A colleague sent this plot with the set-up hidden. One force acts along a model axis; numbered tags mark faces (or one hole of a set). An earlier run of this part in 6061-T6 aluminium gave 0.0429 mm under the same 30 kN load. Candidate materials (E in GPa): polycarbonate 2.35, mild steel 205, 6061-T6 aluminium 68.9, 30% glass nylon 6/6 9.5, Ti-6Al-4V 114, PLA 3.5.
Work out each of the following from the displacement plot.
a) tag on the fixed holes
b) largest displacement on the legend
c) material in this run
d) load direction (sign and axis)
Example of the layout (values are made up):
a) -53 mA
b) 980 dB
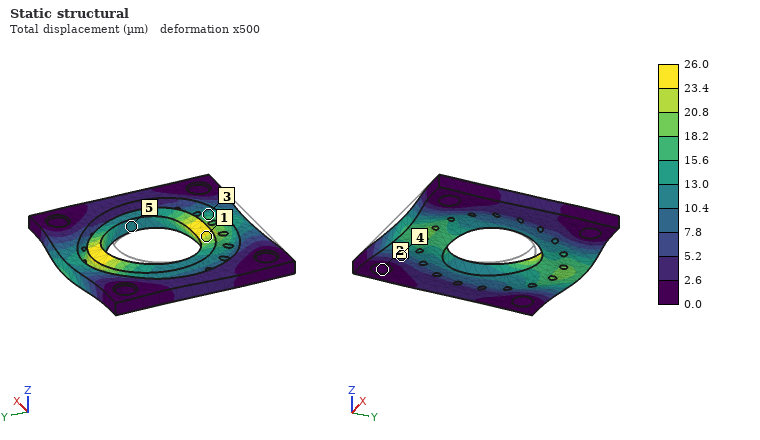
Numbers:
a) 2
b) 26.0 µm
c) Ti-6Al-4V
d) +Y
